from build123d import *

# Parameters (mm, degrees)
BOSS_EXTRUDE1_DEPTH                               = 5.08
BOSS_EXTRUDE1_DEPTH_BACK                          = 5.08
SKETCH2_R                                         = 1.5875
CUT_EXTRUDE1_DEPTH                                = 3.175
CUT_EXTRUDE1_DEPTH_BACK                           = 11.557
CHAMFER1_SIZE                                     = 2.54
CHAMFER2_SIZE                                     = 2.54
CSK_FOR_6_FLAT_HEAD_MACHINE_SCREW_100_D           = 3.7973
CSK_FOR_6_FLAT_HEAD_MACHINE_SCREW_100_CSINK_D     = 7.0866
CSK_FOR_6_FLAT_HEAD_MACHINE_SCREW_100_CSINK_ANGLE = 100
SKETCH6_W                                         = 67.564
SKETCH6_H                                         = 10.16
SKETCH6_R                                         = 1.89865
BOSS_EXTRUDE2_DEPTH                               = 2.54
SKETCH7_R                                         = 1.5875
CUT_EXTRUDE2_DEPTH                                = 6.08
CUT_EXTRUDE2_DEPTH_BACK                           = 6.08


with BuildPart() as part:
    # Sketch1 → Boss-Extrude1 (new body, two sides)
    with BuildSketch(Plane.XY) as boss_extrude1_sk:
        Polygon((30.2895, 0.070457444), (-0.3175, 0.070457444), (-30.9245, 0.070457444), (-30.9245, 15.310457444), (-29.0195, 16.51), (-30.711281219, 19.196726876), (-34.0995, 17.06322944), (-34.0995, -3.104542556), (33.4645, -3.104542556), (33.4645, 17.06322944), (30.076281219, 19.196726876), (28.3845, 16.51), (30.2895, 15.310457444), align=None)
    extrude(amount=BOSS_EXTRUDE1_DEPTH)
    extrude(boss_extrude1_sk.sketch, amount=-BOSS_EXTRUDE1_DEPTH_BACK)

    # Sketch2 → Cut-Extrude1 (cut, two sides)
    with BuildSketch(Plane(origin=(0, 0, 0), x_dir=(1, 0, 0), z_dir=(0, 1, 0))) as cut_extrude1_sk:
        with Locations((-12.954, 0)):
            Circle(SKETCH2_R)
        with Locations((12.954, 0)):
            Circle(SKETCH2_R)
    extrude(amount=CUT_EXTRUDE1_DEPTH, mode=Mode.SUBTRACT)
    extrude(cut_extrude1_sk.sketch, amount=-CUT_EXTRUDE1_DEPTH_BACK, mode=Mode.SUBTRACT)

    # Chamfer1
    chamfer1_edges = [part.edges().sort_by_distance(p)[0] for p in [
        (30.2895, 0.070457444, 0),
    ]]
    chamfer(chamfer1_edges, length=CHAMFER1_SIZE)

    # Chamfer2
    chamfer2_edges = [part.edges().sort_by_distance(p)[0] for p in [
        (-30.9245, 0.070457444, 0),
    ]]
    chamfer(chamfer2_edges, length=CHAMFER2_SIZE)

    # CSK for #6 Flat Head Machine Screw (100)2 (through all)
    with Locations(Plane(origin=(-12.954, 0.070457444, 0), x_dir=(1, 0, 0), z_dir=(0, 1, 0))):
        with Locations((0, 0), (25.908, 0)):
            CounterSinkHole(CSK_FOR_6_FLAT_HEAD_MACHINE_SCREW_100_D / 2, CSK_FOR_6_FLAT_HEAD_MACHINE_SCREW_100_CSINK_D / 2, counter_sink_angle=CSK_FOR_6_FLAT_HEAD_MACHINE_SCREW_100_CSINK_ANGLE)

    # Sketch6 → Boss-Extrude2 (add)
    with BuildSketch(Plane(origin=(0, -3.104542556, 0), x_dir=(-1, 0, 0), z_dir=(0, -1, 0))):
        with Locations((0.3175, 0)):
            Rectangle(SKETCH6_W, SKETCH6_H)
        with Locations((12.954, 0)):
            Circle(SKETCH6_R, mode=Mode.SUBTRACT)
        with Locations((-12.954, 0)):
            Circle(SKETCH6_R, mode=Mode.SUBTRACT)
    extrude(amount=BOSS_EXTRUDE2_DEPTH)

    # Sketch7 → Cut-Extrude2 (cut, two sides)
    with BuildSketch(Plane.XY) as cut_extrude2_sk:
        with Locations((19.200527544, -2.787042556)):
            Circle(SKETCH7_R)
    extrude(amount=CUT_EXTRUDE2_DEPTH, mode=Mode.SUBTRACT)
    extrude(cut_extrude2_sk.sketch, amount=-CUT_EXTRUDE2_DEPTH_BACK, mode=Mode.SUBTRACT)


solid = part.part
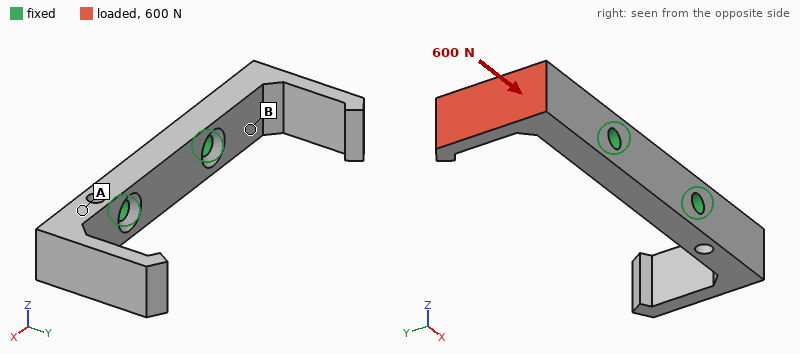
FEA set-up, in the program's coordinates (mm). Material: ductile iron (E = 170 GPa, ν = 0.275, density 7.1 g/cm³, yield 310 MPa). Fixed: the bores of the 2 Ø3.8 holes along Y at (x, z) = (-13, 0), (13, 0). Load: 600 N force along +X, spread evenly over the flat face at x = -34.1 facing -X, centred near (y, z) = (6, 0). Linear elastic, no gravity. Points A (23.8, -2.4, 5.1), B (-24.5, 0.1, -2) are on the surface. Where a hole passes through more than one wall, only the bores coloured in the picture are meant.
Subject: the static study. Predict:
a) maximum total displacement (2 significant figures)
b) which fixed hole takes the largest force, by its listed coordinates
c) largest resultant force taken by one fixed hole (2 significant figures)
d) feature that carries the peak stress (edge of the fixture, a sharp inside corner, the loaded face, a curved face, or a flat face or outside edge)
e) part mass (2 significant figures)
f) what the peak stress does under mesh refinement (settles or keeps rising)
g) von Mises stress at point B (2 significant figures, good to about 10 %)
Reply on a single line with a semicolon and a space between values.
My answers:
0.14 mm; (-13, 0); 530 N; edge of the fixture; 35 g; keeps rising; 100 MPa
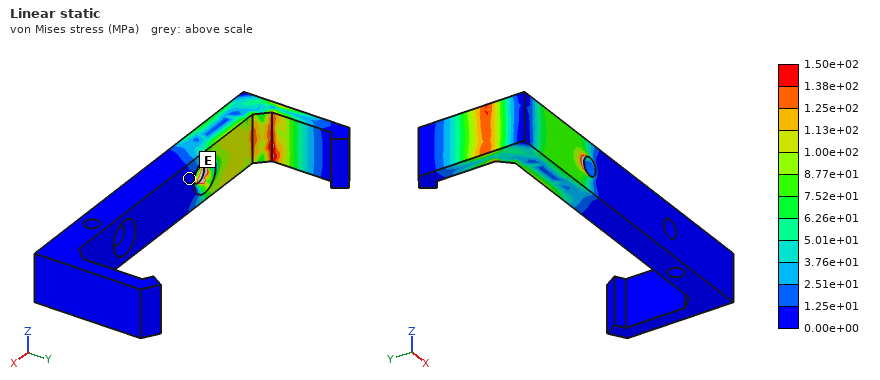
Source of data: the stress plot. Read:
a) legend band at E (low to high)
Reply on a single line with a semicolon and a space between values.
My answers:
0.00e+00 to 1.25e+01 MPa
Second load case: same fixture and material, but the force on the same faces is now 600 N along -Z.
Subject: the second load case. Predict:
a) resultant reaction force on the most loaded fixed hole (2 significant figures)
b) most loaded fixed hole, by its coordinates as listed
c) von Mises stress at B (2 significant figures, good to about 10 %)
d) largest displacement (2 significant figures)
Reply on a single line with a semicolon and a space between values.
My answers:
790 N; (-13, 0); 120 MPa; 0.11 mm
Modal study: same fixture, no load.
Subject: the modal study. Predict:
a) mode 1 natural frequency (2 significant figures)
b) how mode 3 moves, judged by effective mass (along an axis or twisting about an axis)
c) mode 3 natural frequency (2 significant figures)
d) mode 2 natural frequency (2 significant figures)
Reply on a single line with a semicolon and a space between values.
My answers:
4100 Hz; along Z; 5100 Hz; 4100 Hz
